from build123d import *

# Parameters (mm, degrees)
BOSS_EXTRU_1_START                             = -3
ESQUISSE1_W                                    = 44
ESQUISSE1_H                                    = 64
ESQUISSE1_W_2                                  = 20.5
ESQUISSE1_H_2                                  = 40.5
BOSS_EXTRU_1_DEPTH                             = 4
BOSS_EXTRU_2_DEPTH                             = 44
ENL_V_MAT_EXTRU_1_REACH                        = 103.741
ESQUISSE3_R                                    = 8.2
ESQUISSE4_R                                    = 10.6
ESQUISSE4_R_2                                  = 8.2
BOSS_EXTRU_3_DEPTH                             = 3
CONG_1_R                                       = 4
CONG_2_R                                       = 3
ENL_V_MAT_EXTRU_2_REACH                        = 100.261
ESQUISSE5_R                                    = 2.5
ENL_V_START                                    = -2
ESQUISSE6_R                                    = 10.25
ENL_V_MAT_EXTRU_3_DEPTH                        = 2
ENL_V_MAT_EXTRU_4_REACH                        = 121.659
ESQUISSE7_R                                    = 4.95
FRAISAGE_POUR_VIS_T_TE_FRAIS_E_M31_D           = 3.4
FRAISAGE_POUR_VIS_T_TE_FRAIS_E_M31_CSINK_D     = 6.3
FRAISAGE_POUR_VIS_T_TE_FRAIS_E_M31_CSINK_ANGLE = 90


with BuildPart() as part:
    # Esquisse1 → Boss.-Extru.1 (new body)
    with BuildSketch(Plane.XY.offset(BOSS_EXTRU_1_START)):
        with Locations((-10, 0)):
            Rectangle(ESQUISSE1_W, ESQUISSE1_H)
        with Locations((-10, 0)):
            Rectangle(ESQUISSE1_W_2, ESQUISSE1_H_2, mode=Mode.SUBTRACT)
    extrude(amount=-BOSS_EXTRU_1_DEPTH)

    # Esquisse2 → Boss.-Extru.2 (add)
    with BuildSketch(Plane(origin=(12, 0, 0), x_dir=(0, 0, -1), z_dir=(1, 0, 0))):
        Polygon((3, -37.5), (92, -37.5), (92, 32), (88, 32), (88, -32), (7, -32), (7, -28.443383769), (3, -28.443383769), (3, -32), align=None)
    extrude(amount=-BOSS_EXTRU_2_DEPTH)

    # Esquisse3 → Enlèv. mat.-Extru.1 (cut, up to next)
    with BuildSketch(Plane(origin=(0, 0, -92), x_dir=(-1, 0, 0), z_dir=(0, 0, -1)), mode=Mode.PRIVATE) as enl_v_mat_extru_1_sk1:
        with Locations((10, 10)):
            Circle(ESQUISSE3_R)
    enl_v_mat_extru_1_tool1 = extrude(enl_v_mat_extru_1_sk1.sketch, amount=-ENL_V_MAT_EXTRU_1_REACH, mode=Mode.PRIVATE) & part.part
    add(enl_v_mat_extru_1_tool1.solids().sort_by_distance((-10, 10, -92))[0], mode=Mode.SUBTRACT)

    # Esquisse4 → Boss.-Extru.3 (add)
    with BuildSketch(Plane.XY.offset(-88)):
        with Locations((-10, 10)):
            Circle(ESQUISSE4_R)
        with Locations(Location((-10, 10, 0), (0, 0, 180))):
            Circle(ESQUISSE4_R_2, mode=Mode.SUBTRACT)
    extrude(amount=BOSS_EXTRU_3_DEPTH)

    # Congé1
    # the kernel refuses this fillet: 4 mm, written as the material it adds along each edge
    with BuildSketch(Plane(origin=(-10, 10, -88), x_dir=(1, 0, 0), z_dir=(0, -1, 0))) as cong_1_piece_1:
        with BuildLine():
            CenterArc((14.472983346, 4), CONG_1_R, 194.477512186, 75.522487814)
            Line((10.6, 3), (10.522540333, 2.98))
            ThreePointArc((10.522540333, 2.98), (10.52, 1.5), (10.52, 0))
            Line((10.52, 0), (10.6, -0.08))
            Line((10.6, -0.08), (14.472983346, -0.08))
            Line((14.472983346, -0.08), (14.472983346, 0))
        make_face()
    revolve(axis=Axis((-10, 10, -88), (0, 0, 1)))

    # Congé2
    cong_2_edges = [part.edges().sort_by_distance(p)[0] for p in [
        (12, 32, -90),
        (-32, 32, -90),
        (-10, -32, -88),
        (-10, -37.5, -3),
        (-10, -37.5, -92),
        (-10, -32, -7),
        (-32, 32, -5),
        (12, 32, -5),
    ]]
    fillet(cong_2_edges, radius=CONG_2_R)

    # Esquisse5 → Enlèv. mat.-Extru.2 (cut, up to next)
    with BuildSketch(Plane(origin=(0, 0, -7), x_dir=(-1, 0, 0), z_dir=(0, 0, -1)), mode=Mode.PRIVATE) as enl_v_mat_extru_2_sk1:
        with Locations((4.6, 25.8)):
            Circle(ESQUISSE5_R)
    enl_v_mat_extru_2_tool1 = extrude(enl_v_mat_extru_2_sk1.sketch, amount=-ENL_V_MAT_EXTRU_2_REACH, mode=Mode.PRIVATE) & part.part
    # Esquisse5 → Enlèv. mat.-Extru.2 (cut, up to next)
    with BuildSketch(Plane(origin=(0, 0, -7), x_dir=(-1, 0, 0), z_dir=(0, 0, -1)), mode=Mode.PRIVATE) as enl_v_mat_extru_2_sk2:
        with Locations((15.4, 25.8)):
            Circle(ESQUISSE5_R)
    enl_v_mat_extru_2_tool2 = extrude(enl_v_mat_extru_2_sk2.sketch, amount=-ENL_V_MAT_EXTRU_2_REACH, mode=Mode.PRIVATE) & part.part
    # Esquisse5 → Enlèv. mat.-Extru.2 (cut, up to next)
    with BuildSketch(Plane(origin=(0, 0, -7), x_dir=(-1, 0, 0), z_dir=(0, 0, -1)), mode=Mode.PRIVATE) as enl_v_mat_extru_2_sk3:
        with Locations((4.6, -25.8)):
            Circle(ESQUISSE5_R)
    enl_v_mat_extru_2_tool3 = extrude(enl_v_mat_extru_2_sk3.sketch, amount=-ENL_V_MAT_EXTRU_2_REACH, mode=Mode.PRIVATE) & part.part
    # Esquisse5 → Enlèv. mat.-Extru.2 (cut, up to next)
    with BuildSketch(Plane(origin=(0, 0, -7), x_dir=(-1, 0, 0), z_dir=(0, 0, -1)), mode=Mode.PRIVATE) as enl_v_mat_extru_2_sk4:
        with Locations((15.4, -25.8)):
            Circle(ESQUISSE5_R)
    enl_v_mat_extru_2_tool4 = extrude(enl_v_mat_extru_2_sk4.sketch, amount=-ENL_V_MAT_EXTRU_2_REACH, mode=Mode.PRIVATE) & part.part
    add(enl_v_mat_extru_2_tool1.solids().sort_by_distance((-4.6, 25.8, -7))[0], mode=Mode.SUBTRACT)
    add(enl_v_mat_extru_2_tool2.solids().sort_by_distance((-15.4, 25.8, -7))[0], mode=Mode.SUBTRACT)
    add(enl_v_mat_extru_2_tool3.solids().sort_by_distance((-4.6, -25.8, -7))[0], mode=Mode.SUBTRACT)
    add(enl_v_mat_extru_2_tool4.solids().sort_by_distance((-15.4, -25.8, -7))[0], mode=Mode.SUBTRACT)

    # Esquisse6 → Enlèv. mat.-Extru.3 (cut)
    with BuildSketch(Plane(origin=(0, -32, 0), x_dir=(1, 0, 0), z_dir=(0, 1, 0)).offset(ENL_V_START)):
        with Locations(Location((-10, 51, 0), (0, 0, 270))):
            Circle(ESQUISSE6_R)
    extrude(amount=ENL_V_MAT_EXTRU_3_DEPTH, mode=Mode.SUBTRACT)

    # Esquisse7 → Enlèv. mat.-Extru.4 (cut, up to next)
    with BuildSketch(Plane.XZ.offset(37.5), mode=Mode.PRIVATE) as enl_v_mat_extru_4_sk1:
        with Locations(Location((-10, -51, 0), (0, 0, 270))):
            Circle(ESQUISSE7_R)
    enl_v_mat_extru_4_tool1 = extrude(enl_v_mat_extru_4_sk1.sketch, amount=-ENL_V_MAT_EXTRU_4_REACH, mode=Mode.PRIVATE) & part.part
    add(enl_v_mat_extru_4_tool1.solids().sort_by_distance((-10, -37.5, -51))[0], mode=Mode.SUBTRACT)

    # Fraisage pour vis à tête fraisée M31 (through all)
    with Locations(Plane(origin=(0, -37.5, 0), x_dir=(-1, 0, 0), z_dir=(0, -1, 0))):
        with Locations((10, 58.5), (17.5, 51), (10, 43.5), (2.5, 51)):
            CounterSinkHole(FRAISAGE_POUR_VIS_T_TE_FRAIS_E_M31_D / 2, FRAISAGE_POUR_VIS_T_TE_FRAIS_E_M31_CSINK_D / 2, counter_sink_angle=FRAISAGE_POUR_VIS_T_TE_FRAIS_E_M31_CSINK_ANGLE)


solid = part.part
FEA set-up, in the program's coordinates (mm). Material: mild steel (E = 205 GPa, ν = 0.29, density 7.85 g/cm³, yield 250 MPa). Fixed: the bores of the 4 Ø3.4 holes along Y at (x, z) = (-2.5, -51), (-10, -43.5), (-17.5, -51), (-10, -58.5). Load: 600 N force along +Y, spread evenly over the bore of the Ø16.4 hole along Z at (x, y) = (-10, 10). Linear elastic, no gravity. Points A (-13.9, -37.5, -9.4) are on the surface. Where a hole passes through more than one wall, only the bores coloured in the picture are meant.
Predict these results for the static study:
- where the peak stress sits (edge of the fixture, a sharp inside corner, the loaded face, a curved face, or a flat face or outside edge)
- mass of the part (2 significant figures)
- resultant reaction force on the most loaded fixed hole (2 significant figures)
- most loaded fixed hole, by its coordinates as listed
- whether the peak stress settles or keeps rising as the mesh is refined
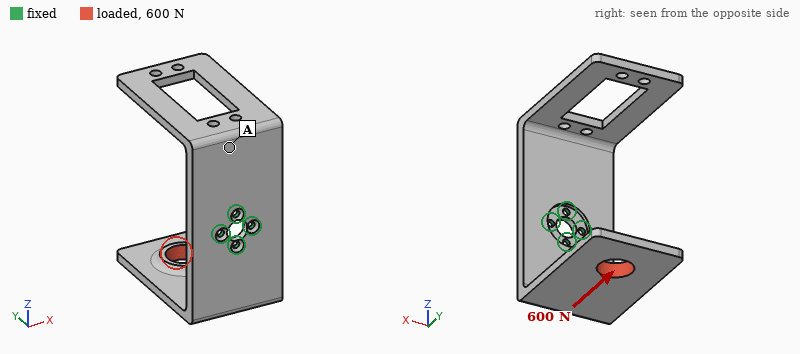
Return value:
edge of the fixture
310 g
1.4 kN
(-10, -58.5)
keeps rising
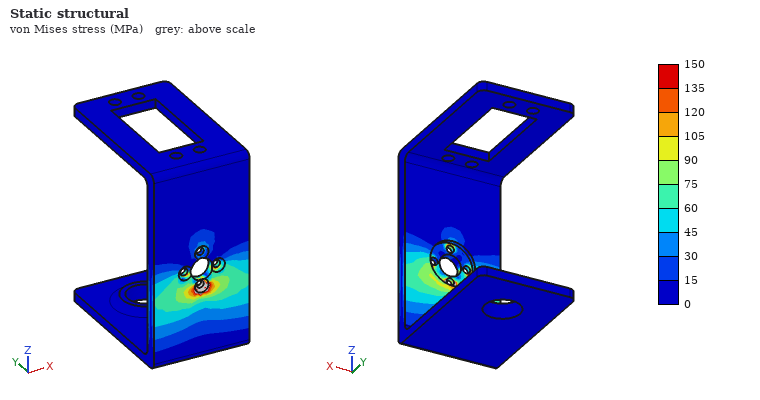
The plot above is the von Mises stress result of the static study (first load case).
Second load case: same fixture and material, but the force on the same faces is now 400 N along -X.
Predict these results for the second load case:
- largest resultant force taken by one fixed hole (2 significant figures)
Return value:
900 N
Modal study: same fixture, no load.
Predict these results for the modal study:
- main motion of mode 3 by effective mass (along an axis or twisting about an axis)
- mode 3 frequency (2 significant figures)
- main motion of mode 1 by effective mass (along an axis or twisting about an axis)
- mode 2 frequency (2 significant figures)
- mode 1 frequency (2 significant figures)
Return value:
along X
860 Hz
along Z
540 Hz
520 Hz
